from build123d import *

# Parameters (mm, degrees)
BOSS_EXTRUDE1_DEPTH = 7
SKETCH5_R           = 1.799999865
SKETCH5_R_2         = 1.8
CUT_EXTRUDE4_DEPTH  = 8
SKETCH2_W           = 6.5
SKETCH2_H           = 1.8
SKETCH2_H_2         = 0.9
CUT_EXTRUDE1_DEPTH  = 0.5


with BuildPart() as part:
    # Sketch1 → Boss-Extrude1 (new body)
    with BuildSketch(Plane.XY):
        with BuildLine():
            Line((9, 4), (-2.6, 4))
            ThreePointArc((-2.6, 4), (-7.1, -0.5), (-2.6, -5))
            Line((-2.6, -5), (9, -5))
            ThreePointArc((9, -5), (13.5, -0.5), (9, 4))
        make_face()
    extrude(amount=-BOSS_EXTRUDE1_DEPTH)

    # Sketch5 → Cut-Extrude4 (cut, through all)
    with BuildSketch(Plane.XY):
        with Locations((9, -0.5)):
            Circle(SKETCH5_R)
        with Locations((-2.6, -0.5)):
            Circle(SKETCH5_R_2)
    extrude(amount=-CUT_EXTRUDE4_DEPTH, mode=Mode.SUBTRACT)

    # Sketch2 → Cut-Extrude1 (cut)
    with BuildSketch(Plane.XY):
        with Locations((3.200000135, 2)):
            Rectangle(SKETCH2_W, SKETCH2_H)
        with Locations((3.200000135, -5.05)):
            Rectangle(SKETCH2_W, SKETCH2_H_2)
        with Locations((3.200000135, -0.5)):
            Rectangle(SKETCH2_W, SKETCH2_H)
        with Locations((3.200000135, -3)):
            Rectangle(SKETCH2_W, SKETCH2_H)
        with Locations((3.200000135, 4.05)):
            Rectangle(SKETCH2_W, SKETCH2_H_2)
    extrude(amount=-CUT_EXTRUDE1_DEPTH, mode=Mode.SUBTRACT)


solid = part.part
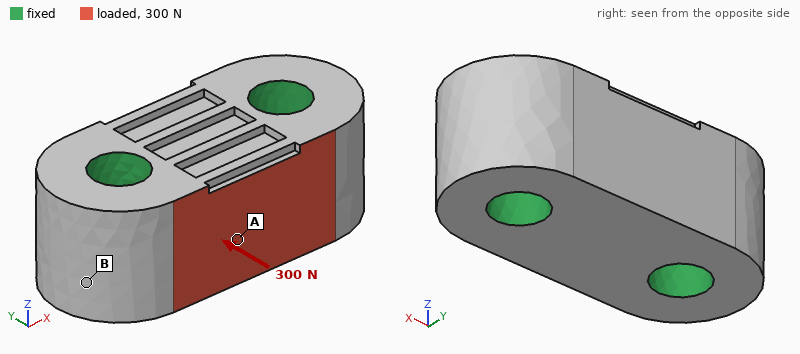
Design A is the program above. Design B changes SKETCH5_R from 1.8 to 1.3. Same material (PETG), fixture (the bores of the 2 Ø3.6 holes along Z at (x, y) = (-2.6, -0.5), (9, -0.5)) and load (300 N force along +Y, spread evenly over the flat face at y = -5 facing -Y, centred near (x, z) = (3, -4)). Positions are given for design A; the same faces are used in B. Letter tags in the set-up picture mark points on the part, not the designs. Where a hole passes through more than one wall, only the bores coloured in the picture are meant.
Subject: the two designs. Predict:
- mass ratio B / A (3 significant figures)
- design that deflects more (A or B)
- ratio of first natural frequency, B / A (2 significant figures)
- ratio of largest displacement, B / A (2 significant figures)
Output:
1.03
B
0.92
1.1
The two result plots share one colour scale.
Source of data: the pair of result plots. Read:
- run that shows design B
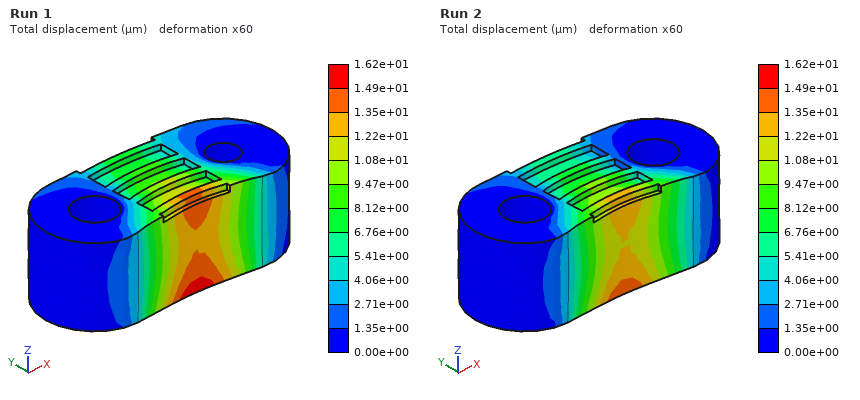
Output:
Run 1
